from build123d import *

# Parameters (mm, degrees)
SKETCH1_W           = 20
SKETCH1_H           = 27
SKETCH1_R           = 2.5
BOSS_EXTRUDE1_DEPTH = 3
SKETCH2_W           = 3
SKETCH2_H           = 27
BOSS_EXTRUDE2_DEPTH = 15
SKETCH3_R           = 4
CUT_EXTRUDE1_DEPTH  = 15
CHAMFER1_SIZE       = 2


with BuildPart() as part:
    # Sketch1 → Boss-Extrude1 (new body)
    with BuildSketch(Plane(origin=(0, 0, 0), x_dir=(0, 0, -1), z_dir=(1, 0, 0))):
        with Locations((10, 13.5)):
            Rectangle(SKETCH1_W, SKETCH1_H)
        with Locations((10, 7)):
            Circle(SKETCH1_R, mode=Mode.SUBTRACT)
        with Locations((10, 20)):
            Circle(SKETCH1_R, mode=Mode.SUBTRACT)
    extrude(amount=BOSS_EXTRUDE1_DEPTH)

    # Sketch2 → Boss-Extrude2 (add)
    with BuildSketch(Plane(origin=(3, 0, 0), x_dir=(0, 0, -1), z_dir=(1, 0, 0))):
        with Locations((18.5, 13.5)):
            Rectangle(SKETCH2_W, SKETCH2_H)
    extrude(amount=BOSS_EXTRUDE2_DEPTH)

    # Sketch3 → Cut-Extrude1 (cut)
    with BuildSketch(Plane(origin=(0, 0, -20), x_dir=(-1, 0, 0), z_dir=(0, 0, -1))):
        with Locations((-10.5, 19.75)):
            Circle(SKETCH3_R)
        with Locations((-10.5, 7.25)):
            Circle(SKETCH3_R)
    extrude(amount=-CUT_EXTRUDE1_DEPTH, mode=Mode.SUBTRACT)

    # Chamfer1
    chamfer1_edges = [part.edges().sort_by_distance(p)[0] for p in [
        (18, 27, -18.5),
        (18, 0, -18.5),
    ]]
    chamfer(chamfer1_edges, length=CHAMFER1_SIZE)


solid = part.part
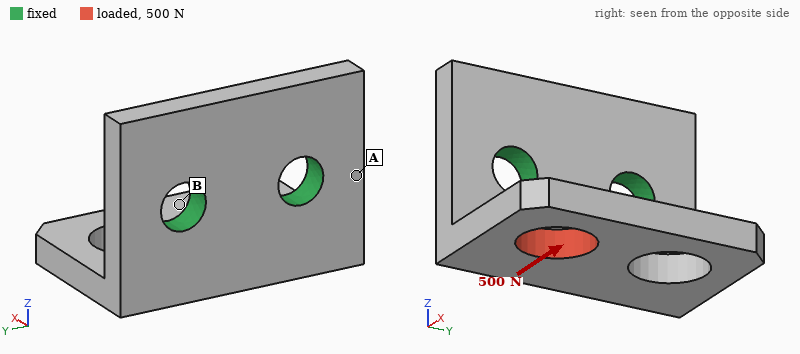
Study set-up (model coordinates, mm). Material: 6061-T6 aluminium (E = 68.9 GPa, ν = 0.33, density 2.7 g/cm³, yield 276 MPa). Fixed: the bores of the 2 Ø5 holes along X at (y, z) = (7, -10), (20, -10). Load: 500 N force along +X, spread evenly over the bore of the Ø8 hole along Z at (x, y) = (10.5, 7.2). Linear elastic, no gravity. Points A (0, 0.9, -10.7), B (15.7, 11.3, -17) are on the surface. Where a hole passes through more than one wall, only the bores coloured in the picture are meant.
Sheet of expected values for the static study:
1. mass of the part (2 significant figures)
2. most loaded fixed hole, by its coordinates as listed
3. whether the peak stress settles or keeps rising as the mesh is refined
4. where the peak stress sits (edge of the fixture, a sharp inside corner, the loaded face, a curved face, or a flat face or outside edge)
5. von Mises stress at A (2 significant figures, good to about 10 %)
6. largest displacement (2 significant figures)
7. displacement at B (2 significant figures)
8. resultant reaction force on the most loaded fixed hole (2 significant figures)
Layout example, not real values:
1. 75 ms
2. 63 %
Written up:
1. 6.5 g
2. (7, -10)
3. keeps rising
4. edge of the fixture
5. 48 MPa
6. 71 µm
7. 49 µm
8. 430 N
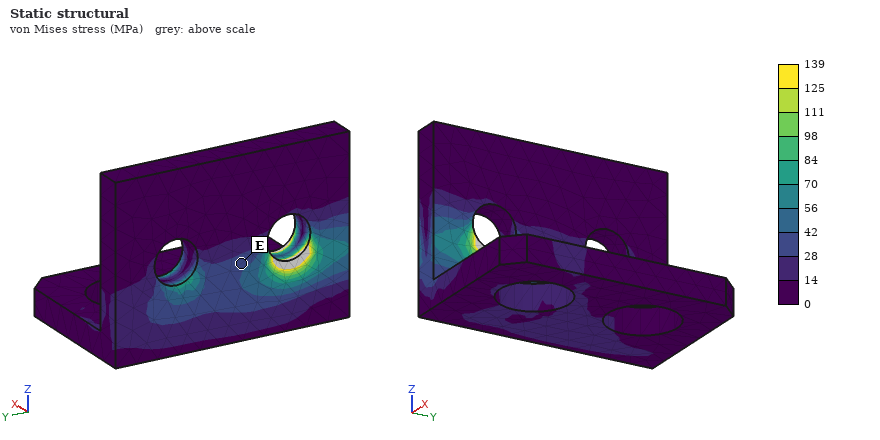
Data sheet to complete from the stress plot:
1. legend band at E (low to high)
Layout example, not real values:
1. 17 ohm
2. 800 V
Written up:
1. 28 to 42 MPa
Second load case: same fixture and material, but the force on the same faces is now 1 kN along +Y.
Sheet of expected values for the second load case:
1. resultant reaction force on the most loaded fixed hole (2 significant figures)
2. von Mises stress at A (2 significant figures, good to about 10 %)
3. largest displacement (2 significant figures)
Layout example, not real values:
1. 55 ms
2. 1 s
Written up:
1. 840 N
2. 72 MPa
3. 82 µm
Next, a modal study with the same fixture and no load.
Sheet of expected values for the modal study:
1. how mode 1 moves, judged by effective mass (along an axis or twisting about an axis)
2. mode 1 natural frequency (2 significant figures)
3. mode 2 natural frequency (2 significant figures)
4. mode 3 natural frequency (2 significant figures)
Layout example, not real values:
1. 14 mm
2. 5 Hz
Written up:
1. along Z
2. 5900 Hz
3. 10 kHz
4. 15 kHz
